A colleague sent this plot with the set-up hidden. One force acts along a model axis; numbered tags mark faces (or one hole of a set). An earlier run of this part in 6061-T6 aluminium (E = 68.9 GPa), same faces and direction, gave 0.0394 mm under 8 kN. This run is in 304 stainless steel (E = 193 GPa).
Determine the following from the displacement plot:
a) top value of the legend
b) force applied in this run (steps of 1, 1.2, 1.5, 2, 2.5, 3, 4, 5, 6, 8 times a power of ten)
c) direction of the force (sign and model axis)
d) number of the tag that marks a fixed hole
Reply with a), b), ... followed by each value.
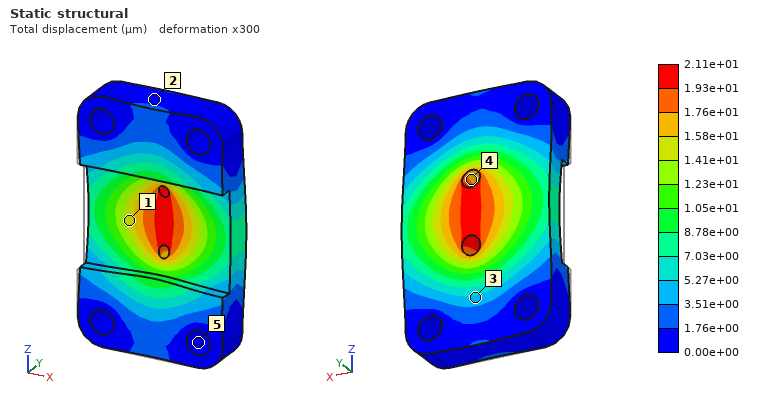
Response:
a) 2.11e+01 µm
b) 12 kN
c) +Y
d) 5
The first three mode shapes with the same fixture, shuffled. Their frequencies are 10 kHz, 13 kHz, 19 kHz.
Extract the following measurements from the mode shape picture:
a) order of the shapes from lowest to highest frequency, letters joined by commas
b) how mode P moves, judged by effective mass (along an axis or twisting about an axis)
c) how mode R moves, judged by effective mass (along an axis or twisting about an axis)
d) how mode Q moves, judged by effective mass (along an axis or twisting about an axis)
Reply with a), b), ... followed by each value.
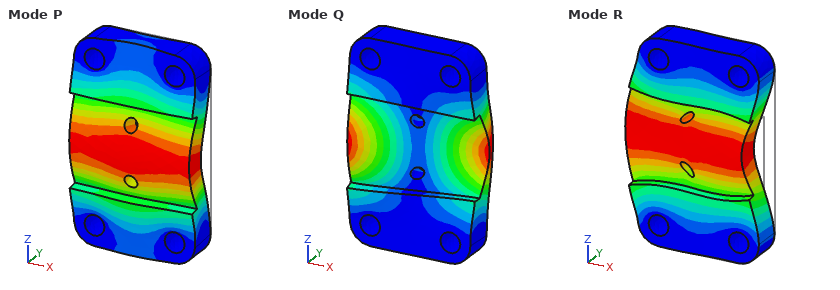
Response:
a) P, Q, R
b) along Y
c) along X
d) twisting about Z
